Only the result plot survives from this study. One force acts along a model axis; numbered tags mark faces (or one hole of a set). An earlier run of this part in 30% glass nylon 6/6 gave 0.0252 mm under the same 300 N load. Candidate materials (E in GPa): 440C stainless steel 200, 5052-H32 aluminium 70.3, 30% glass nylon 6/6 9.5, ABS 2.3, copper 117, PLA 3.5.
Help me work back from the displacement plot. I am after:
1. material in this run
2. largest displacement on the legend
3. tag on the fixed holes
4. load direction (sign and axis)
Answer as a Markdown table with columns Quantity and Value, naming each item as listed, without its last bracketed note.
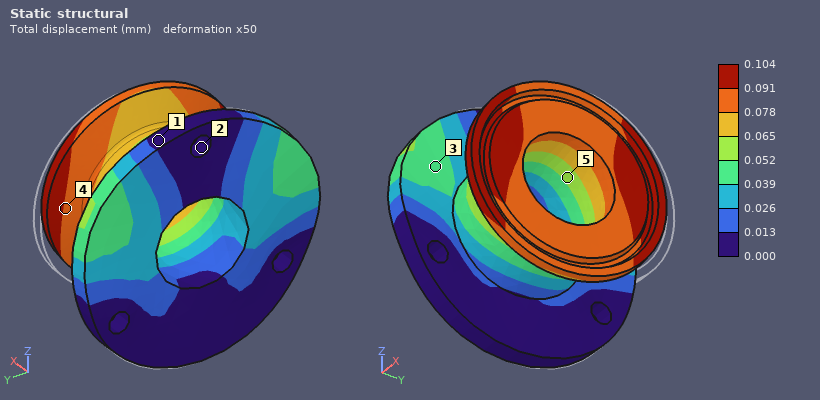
| Quantity | Value |
|---|---|
| material in this run | ABS |
| largest displacement on the legend | 0.104 mm |
| tag on the fixed holes | 2 |
| load direction | -Y |
